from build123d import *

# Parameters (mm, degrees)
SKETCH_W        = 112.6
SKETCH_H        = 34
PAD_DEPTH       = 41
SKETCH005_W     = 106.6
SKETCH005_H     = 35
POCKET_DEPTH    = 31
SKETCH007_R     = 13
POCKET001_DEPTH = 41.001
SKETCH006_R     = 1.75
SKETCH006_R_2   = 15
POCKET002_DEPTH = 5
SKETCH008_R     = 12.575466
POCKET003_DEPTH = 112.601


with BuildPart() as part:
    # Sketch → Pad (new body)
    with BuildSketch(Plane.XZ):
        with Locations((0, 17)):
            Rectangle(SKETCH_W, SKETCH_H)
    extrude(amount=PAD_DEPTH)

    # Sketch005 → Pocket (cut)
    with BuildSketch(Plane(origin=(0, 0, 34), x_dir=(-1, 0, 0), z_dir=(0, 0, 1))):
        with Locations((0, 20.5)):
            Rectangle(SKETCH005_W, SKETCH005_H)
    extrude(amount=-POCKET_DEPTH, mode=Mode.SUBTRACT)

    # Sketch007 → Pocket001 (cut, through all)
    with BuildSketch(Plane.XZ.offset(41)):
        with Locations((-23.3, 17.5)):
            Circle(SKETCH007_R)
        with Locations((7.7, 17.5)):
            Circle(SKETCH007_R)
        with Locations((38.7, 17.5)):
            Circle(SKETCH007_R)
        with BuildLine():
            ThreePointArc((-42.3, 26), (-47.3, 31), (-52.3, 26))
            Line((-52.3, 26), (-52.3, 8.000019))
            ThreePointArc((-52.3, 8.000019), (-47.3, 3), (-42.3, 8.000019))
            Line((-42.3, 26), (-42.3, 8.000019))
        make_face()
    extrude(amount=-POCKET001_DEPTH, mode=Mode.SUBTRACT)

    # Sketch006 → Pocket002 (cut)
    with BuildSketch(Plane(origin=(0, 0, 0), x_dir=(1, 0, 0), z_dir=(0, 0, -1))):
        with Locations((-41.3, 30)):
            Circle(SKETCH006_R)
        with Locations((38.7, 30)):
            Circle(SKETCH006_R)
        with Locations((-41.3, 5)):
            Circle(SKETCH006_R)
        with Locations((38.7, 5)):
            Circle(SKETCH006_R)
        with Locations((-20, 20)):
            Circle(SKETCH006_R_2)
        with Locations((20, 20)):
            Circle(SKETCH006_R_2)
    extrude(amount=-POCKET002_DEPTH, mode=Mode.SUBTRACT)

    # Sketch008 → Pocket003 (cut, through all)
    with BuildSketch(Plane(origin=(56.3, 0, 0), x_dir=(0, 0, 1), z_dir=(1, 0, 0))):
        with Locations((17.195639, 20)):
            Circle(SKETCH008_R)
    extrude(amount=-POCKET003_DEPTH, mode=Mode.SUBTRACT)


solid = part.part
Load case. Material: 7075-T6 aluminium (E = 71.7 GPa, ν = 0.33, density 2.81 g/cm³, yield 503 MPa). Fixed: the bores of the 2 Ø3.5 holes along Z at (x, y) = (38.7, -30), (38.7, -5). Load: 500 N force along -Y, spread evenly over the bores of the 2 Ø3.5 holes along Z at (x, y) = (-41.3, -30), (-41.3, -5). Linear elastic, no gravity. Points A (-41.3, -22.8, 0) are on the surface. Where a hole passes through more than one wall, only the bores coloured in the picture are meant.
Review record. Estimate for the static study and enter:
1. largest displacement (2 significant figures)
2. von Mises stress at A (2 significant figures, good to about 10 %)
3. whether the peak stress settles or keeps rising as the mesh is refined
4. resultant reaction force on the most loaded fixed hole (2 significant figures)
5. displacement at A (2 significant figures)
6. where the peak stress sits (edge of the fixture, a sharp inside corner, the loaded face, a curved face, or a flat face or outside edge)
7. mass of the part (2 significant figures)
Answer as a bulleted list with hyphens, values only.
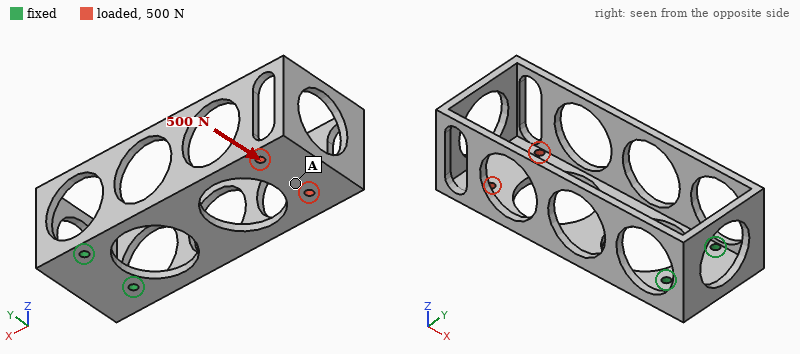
- 0.32 mm
- 14 MPa
- keeps rising
- 1.5 kN
- 0.24 mm
- edge of the fixture
- 64 g
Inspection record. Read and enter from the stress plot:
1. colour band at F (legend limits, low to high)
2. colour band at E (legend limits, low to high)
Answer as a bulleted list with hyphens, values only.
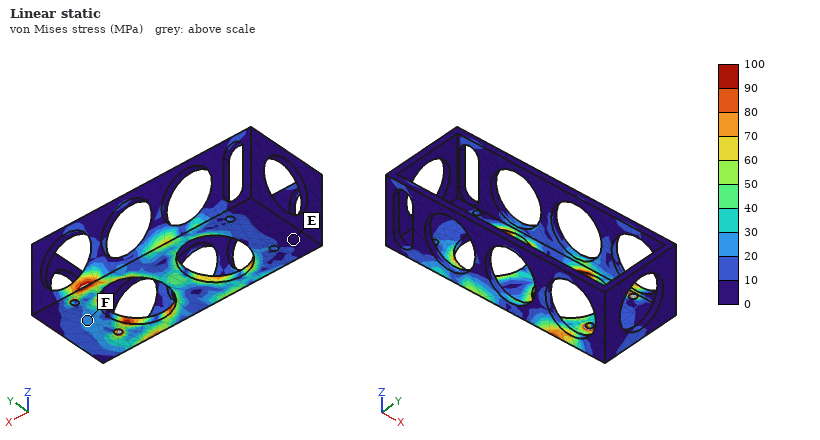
- 20 to 30 MPa
- 0 to 10 MPa
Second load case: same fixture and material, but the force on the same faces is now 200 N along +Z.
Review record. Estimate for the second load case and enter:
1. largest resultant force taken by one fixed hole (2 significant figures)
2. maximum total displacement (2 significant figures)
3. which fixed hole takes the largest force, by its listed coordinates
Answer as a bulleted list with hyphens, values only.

- 160 N
- 1.1 mm
- (38.7, -5)
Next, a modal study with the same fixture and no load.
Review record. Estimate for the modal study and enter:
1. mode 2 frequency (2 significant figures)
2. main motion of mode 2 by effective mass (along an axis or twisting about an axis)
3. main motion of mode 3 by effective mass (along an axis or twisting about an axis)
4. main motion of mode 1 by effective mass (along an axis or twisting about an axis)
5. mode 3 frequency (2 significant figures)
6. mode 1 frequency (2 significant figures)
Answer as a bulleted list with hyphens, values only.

- 700 Hz
- along Y
- along Y
- along Z
- 1600 Hz
- 420 Hz
